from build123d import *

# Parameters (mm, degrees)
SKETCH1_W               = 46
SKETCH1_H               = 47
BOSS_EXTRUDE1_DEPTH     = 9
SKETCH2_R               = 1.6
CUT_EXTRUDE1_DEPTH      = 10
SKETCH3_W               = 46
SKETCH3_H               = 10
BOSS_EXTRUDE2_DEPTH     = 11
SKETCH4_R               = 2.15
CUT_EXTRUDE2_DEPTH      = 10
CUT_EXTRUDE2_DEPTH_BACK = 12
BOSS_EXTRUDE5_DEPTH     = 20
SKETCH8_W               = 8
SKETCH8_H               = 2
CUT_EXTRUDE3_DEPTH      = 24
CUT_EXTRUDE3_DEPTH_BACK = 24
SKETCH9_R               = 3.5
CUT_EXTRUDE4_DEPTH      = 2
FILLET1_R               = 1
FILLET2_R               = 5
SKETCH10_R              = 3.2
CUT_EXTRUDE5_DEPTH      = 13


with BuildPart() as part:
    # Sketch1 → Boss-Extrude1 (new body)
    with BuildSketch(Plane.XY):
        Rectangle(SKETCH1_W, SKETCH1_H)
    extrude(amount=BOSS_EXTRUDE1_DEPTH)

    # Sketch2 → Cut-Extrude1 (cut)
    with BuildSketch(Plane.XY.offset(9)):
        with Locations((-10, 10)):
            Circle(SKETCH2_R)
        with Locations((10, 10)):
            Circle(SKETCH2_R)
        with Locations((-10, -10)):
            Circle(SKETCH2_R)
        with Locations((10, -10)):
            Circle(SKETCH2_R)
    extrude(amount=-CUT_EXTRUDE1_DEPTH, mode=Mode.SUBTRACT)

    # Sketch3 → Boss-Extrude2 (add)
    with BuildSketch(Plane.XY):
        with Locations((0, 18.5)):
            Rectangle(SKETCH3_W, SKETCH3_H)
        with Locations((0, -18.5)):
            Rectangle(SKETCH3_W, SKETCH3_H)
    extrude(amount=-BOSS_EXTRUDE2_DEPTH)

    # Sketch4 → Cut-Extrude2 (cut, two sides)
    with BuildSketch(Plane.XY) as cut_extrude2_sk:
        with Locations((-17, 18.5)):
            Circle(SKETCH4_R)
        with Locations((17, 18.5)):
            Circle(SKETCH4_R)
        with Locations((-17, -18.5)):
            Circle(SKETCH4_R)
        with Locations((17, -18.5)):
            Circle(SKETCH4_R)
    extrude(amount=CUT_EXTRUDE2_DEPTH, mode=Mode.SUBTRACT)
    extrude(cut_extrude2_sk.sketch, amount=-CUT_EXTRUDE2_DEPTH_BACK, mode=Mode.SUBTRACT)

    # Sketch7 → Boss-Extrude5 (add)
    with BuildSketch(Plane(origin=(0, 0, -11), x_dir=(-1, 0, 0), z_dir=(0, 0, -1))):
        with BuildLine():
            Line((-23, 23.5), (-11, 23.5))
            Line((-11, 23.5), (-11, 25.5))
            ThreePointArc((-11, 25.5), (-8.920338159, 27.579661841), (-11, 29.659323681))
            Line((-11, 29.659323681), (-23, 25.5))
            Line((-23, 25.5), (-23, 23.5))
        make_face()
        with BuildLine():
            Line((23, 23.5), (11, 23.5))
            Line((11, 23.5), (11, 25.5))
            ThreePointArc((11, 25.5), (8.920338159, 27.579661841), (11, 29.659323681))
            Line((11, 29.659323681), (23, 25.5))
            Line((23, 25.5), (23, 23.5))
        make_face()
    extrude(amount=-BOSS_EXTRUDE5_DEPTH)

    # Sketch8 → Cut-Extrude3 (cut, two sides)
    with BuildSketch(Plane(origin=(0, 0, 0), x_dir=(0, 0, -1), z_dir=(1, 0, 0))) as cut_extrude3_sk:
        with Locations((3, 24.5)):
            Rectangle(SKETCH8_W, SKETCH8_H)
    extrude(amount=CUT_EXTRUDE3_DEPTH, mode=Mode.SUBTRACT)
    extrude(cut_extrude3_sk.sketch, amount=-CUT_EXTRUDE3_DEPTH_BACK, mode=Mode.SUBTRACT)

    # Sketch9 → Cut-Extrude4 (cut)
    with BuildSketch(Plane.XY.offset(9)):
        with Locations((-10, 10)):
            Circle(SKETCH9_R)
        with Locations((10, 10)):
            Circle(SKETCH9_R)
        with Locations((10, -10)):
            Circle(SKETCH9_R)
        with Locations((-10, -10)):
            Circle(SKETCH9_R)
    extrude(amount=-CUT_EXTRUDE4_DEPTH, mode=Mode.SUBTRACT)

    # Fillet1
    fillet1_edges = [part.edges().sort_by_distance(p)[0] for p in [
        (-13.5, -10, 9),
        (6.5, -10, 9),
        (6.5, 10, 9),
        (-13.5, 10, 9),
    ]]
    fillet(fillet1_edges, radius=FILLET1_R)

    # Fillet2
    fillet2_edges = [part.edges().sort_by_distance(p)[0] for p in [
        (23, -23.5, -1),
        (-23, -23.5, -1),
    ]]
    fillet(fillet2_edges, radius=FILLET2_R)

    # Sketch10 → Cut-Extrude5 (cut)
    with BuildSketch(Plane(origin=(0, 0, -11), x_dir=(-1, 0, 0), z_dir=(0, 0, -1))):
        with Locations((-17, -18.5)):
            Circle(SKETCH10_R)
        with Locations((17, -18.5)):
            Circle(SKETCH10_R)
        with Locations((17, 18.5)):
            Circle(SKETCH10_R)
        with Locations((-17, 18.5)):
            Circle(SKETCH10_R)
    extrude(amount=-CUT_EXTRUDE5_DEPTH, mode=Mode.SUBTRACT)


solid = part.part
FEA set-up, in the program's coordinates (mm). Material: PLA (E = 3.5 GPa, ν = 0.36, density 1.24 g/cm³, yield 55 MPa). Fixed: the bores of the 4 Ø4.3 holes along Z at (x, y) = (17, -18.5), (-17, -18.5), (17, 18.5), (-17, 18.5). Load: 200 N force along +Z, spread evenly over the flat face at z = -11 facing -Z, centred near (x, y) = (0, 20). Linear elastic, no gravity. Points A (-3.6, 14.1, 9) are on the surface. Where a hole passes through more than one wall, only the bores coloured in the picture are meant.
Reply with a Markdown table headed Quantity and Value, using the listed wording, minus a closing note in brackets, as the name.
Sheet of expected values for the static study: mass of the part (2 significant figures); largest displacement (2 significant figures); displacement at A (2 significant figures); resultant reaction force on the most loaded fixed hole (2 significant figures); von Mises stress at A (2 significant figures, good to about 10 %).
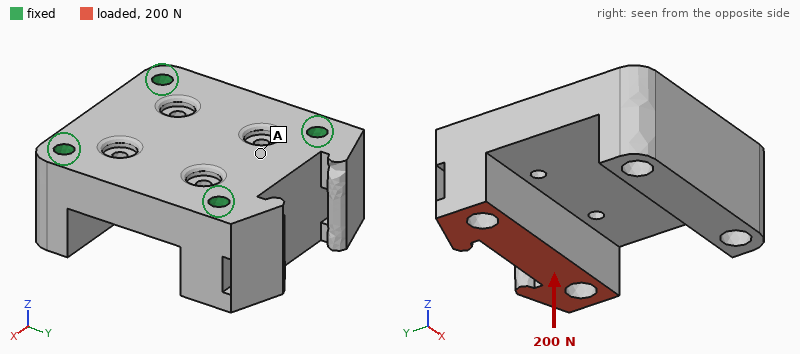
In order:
| Quantity | Value |
|---|---|
| mass of the part | 35 g |
| largest displacement | 8.8 µm |
| displacement at A | 3.5 µm |
| resultant reaction force on the most loaded fixed hole | 100 N |
| von Mises stress at A | 0.33 MPa |
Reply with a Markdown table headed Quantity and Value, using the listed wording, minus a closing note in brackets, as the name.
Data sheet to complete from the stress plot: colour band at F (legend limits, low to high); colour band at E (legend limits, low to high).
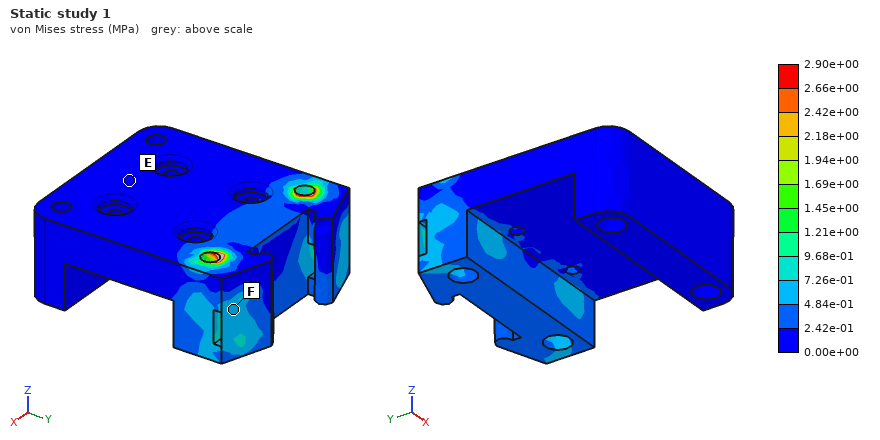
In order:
| Quantity | Value |
|---|---|
| colour band at F | 4.84e-01 to 7.26e-01 MPa |
| colour band at E | 0.00e+00 to 2.42e-01 MPa |
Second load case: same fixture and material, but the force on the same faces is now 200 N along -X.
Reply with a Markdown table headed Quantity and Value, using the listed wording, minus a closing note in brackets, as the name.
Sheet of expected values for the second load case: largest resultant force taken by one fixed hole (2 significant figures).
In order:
| Quantity | Value |
|---|---|
| largest resultant force taken by one fixed hole | 120 N |
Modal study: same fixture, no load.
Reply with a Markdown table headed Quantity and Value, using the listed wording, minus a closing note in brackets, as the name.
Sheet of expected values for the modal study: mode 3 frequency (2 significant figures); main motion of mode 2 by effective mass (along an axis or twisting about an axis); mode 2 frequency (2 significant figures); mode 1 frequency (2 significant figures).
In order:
| Quantity | Value |
|---|---|
| mode 3 frequency | 7700 Hz |
| main motion of mode 2 by effective mass | along Y |
| mode 2 frequency | 6300 Hz |
| mode 1 frequency | 5100 Hz |
